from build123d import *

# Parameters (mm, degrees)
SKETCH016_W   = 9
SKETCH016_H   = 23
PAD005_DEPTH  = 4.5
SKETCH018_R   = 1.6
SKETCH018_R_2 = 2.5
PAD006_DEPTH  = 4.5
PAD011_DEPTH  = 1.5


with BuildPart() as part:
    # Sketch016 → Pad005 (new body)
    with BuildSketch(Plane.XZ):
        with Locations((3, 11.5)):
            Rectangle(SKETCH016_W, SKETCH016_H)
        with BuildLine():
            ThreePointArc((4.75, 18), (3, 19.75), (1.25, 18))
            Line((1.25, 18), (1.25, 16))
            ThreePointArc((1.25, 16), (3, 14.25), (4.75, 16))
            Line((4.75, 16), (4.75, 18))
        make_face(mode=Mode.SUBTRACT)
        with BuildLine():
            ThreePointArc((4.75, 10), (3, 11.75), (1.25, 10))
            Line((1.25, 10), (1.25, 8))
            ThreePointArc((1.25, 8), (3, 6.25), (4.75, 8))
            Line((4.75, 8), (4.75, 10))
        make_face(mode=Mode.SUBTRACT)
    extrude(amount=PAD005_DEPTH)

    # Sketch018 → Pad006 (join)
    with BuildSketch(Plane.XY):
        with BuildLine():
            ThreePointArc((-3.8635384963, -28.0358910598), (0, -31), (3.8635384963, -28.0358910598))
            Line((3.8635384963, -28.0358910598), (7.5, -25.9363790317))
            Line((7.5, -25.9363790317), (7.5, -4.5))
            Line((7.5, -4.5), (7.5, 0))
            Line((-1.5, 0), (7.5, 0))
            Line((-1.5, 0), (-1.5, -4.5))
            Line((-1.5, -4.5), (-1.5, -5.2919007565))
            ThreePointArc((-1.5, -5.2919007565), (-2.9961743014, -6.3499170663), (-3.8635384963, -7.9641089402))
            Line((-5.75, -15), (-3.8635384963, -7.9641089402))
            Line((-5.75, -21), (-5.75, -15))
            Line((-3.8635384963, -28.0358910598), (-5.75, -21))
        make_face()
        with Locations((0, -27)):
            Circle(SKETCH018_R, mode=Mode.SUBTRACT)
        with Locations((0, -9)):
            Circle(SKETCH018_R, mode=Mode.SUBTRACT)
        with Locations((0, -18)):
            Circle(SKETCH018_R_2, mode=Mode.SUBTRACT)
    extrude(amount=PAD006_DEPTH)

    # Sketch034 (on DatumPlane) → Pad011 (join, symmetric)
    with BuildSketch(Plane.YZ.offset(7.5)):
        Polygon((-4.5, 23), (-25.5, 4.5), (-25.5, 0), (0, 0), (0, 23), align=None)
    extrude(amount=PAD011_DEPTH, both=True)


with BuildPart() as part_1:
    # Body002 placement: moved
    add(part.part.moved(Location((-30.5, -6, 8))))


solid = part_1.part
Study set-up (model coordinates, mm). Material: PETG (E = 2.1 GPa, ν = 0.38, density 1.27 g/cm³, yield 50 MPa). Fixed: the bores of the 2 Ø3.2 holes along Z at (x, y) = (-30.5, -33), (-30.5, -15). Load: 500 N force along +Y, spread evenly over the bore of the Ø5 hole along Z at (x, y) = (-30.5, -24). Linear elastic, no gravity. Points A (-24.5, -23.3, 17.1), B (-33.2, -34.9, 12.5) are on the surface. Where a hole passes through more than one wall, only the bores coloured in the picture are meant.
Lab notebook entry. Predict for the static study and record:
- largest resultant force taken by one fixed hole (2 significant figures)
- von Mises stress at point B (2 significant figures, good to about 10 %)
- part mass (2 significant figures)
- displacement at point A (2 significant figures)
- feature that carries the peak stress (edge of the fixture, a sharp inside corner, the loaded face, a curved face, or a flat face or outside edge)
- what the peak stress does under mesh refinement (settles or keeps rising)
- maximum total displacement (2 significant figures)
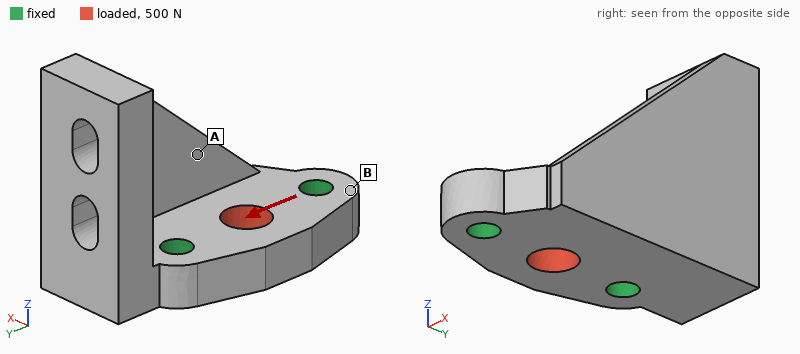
250 N
2.6 MPa
3.6 g
13 µm
edge of the fixture
keeps rising
29 µm
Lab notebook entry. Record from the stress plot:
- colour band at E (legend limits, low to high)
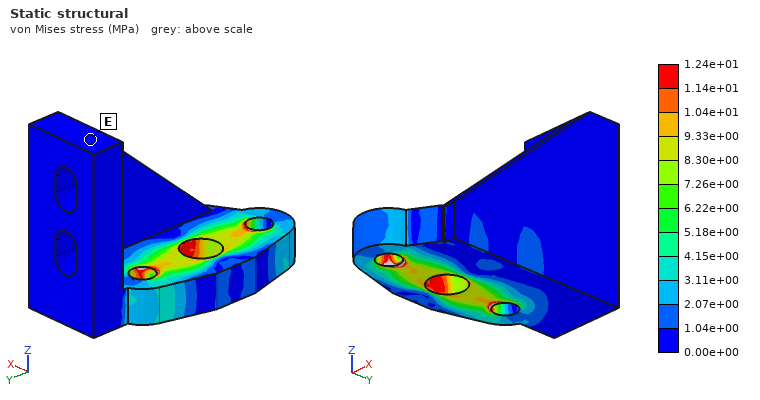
0.00e+00 to 1.04e+00 MPa
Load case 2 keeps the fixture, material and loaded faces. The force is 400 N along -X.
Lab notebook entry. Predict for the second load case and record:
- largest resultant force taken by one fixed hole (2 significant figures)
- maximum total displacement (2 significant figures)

200 N
58 µm
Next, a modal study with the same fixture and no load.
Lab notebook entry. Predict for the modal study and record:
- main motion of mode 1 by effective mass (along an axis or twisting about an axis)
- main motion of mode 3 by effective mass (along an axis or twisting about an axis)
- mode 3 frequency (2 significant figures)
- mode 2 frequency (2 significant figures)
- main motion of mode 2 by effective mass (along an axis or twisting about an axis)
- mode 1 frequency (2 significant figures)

along X
along Z
5500 Hz
3200 Hz
along Y
1800 Hz
